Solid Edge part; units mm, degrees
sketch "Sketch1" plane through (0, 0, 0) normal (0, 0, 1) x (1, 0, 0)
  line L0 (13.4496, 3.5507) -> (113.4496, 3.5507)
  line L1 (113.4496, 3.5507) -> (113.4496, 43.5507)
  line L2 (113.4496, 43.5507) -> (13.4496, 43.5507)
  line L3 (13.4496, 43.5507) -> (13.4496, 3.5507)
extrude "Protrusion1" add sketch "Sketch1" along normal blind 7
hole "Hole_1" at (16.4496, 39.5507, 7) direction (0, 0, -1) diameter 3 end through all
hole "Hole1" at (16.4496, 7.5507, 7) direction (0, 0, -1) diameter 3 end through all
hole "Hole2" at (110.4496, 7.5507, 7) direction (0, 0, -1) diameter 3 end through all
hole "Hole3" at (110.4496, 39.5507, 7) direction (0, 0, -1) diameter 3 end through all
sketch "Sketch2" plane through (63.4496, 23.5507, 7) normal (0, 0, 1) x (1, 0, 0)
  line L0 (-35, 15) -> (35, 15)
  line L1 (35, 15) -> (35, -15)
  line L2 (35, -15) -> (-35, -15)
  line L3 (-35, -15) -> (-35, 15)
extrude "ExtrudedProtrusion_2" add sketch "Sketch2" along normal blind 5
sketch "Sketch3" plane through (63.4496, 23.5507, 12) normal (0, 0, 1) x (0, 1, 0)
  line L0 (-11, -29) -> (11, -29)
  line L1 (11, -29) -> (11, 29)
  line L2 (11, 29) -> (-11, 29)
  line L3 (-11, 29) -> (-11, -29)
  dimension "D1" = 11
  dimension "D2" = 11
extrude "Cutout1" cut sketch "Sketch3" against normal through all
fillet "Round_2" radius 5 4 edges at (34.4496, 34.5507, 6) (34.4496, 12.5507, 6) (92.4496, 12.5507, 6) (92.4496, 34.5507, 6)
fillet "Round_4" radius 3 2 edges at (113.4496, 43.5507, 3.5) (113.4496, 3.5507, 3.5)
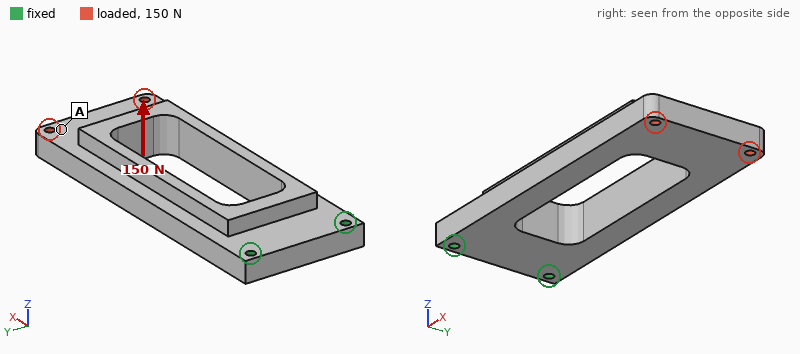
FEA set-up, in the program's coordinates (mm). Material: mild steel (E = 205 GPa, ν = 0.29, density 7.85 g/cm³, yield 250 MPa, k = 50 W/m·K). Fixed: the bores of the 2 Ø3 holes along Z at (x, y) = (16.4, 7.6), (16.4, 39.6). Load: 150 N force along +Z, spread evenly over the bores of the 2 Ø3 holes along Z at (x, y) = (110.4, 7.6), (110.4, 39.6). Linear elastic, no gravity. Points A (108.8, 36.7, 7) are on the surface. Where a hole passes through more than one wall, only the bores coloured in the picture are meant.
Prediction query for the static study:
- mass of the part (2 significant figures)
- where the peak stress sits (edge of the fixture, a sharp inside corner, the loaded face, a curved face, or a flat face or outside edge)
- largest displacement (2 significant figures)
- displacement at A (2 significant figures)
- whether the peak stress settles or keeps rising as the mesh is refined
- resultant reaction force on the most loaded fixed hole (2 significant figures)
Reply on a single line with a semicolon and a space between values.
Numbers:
180 g; edge of the fixture; 0.19 mm; 0.17 mm; keeps rising; 120 N
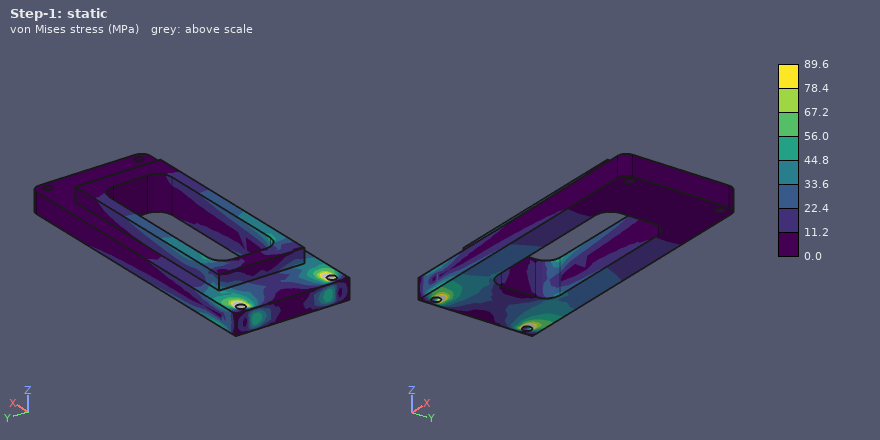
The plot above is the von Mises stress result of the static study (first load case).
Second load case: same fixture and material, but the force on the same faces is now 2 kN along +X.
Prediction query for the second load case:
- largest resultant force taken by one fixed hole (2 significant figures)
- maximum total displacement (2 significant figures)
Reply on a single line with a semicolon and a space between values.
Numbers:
1.0 kN; 29 µm
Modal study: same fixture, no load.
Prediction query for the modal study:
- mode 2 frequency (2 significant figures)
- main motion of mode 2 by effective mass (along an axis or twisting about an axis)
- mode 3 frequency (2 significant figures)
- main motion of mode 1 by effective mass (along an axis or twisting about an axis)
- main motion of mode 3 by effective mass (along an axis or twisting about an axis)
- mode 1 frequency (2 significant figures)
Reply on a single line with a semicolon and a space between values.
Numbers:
1500 Hz; along Y; 2300 Hz; along Z; twisting about X; 620 Hz
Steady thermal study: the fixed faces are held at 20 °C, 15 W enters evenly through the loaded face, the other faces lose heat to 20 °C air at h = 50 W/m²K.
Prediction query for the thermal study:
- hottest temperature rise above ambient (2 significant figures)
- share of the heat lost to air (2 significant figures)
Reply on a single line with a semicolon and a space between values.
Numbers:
67 K; 80 %
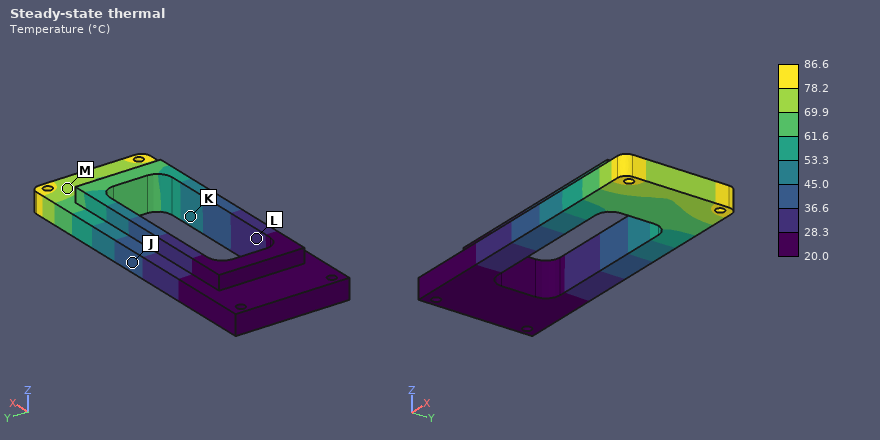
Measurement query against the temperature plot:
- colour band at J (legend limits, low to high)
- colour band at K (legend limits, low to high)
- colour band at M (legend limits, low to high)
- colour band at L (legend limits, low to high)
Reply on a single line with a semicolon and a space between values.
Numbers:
36.6 to 45.0 °C; 45.0 to 53.3 °C; 69.9 to 78.2 °C; 28.3 to 36.6 °C
